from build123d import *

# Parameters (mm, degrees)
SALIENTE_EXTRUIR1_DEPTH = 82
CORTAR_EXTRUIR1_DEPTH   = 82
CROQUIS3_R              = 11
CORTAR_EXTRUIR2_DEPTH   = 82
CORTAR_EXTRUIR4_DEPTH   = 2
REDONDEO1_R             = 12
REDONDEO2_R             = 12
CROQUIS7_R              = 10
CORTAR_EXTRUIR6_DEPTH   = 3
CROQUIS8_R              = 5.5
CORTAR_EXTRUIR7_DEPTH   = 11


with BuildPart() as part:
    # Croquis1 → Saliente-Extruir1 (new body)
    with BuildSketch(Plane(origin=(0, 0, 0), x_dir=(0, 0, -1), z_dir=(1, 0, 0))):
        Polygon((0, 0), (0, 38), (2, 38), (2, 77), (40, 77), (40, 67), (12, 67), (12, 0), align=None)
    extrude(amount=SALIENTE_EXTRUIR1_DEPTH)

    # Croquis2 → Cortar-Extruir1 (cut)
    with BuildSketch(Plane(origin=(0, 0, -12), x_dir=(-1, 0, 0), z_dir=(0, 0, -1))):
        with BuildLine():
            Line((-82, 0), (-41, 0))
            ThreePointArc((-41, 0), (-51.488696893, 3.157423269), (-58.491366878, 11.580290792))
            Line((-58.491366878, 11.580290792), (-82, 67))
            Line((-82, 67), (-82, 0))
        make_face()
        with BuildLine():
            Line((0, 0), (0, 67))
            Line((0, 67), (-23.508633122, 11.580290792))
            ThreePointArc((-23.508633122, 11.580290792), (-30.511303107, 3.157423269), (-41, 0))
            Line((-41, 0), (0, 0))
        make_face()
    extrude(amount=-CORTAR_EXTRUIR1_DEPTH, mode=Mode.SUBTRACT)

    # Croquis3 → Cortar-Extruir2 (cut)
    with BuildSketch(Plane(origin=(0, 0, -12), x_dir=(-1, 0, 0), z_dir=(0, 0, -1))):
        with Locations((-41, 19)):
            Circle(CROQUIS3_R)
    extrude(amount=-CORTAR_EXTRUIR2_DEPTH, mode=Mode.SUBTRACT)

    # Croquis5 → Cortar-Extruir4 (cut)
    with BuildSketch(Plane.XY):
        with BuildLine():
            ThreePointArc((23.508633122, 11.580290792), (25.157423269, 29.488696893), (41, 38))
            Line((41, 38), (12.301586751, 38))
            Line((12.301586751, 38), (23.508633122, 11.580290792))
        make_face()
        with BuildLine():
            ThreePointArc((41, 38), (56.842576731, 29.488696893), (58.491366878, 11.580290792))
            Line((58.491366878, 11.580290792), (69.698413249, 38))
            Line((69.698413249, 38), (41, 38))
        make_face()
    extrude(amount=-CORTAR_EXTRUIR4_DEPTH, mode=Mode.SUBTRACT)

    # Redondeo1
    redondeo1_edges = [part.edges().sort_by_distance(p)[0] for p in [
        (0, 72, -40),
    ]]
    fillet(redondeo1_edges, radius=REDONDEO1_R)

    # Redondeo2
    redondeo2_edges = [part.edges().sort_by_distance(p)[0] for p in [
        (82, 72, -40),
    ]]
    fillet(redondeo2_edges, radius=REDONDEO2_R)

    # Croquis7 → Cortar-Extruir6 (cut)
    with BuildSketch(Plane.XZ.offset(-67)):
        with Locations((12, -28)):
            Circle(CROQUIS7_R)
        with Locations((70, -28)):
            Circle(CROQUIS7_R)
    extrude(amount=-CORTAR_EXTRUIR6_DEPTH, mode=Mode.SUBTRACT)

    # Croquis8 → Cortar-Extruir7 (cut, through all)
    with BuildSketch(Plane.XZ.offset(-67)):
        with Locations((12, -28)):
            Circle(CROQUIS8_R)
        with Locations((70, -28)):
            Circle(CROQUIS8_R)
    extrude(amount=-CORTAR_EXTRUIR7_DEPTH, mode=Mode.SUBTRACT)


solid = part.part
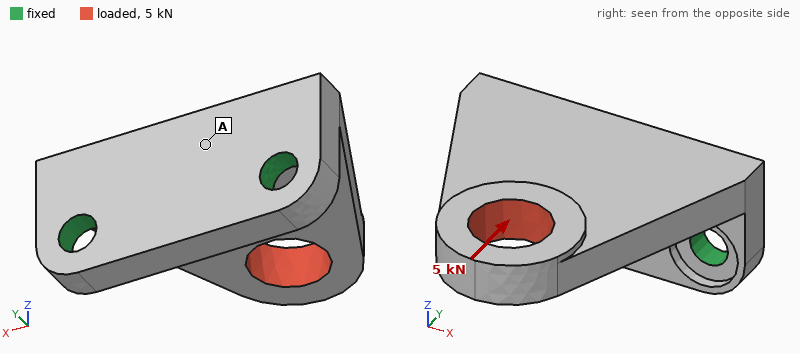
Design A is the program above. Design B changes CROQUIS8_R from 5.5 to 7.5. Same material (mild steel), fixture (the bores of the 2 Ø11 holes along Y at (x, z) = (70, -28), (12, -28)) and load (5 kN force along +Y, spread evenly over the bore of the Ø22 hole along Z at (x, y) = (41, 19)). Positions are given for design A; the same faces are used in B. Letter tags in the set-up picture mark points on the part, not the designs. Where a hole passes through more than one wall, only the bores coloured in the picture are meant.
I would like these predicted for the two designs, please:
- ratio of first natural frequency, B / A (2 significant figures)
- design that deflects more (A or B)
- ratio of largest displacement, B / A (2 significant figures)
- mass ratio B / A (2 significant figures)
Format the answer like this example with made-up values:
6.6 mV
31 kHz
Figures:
1.1
A
0.73
0.98
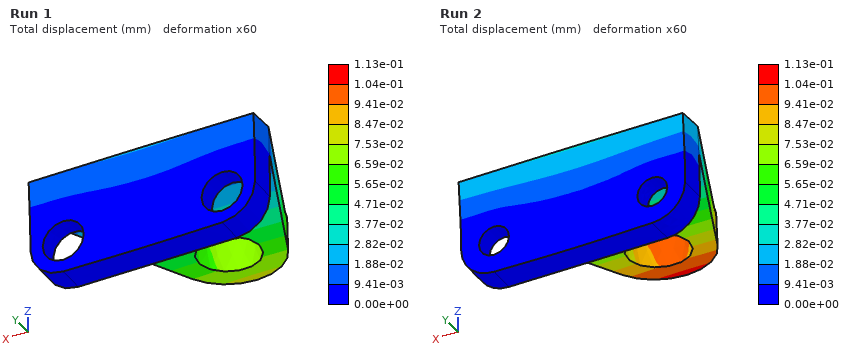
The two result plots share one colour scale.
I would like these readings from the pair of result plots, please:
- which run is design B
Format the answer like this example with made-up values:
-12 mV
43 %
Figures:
Run 1
